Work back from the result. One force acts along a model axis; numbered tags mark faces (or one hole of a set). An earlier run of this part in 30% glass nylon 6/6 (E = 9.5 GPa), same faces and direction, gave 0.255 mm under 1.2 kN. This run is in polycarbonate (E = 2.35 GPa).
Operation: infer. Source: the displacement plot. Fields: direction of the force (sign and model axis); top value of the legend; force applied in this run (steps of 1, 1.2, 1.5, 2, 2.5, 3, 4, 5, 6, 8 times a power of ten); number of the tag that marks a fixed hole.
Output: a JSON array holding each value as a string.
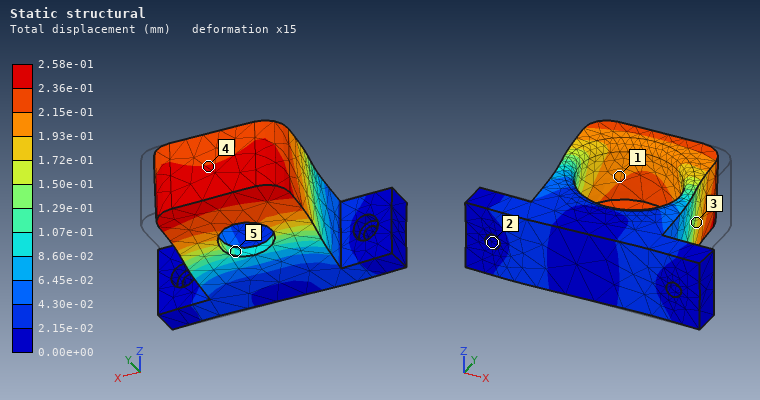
["-X", "2.58e-01 mm", "300 N", "2"]
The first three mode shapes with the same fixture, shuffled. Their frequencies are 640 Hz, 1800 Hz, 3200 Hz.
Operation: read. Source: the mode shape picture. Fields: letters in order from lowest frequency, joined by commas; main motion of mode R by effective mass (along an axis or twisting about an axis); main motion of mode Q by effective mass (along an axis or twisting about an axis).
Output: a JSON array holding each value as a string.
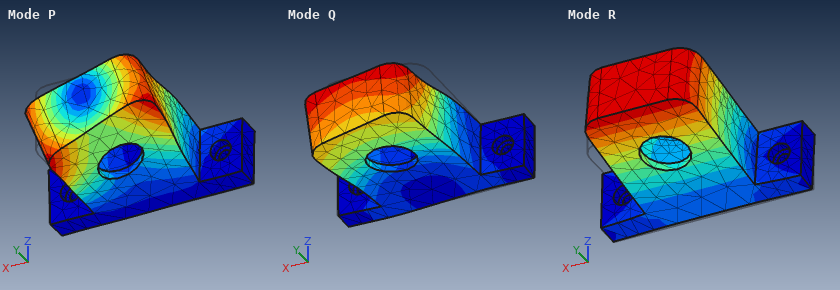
["R, Q, P", "along Z", "along X"]
